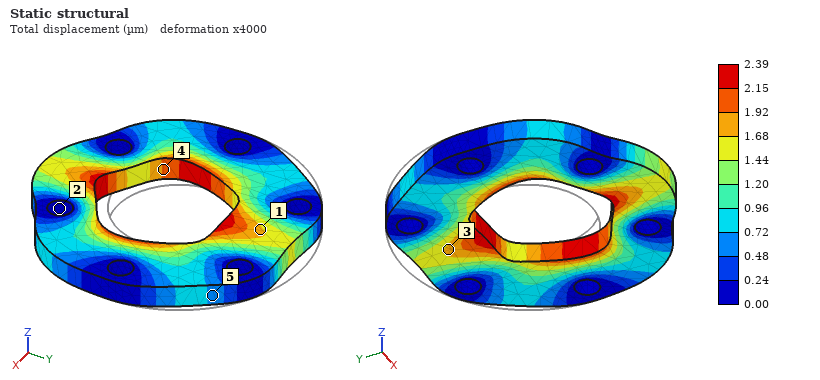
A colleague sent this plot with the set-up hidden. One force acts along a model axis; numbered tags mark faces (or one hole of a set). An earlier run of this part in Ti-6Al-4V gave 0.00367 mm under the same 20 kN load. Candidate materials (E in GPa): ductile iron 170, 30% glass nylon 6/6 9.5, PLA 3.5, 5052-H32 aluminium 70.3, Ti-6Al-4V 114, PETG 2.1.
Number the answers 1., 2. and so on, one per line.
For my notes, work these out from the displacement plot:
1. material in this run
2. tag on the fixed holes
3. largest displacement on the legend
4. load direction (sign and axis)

1. ductile iron
2. 2
3. 2.39 µm
4. -Y
